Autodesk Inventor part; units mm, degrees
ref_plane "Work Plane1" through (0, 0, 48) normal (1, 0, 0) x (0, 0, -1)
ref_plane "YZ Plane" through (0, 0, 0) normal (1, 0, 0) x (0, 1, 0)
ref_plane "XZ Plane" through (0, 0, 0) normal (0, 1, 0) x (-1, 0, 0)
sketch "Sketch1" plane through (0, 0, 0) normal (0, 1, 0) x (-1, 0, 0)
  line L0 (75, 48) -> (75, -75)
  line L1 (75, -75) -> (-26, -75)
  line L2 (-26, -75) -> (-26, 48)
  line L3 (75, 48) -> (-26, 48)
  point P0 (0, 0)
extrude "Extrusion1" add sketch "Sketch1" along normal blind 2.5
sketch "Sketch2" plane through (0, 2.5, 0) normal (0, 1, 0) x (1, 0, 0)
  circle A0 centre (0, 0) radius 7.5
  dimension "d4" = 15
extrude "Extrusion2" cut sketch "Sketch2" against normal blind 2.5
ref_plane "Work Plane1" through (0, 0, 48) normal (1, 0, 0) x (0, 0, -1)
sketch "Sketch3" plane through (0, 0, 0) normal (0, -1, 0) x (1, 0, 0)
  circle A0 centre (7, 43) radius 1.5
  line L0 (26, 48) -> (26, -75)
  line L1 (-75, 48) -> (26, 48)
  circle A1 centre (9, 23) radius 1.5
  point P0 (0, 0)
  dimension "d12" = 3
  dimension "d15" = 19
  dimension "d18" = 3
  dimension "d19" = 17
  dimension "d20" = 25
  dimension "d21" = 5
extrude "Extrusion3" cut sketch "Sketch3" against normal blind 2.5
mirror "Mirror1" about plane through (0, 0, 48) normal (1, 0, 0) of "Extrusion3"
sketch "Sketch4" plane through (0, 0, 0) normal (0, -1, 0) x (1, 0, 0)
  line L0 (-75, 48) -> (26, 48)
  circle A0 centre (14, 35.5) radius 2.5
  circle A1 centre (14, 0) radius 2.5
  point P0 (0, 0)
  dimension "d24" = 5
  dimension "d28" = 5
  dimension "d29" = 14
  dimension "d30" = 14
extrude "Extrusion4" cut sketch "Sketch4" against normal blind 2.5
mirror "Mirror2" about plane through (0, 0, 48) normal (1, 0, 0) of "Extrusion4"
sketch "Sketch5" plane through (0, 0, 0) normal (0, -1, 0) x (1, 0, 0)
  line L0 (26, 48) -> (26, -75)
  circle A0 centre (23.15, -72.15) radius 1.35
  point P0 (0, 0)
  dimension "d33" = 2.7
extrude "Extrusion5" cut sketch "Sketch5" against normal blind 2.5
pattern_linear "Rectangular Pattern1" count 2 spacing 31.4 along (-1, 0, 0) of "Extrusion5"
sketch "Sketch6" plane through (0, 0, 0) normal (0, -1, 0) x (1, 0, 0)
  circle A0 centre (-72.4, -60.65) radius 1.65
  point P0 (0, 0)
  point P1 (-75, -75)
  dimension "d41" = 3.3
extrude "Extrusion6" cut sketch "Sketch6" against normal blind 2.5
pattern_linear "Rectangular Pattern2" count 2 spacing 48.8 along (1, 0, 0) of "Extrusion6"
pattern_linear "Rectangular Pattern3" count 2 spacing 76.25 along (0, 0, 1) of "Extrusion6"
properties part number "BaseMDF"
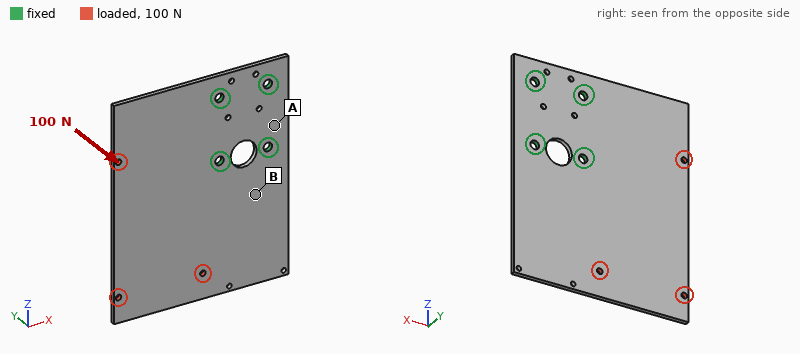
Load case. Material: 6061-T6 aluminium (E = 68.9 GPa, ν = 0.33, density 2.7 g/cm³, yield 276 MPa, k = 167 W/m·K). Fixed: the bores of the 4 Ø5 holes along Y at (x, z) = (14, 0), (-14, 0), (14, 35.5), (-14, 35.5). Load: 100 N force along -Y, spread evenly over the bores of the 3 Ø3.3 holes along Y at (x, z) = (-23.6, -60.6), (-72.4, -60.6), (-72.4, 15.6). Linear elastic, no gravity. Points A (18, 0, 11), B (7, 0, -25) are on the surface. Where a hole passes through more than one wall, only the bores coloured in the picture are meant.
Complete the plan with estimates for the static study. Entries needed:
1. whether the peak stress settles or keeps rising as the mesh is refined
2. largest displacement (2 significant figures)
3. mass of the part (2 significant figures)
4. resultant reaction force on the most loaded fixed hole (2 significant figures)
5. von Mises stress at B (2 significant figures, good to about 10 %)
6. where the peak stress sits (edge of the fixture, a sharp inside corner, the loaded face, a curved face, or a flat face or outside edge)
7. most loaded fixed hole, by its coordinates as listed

keeps rising
1.7 mm
82 g
180 N
29 MPa
edge of the fixture
(-14, 0)
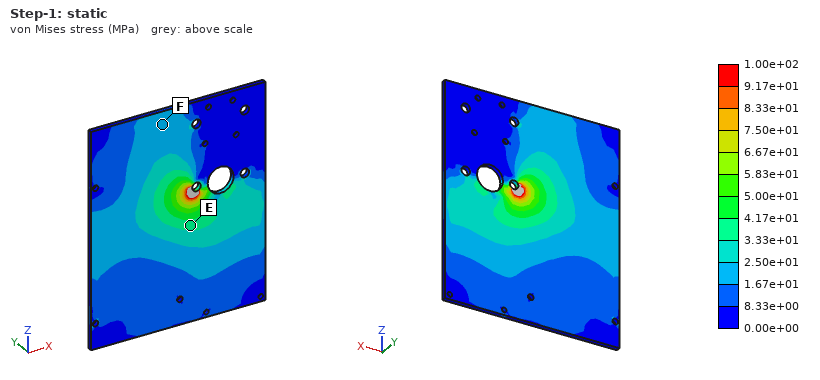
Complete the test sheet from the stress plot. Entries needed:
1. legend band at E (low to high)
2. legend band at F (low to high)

3.33e+01 to 4.17e+01 MPa
1.67e+01 to 2.50e+01 MPa
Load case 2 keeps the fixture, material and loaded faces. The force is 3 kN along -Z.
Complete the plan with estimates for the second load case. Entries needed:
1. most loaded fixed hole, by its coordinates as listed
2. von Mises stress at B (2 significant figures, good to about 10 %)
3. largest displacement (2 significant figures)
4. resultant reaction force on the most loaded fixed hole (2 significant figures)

(-14, 0)
15 MPa
0.12 mm
3.2 kN
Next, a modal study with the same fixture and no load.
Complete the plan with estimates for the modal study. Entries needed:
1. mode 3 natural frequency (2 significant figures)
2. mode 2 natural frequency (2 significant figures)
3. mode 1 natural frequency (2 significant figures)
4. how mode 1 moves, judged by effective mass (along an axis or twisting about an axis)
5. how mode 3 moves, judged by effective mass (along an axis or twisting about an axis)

780 Hz
480 Hz
300 Hz
along Y
along Y
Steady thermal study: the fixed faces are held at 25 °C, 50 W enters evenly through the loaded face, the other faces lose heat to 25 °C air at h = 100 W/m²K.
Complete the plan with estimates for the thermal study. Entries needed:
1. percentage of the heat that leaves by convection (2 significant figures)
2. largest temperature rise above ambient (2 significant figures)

72 %
62 K
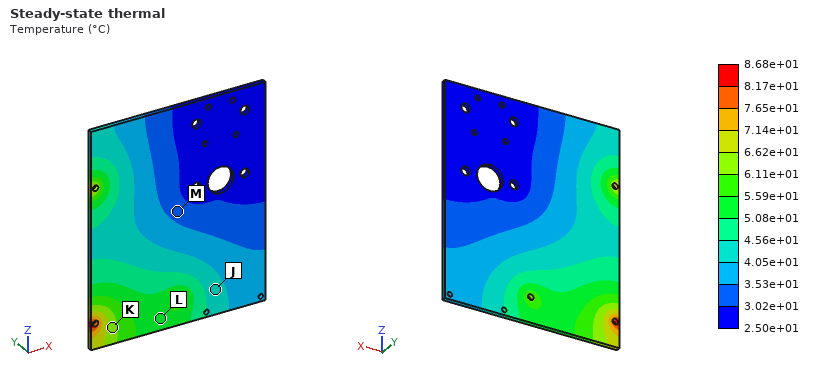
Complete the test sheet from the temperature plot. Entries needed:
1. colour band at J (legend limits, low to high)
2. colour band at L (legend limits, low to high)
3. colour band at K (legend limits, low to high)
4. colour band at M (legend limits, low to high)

4.05e+01 to 4.56e+01 °C
5.08e+01 to 5.59e+01 °C
6.11e+01 to 6.62e+01 °C
3.02e+01 to 3.53e+01 °C
